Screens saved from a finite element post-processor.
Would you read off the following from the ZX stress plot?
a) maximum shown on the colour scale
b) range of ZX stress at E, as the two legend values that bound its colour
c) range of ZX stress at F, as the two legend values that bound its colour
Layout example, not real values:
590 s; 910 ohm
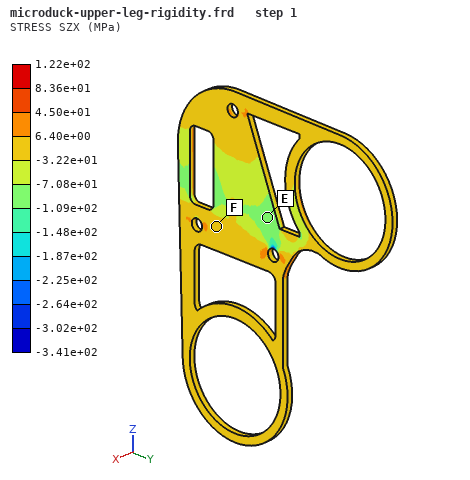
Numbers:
1.22e+02 MPa; -1.09e+02 to -7.08e+01 MPa; -3.22e+01 to 6.40e+00 MPa
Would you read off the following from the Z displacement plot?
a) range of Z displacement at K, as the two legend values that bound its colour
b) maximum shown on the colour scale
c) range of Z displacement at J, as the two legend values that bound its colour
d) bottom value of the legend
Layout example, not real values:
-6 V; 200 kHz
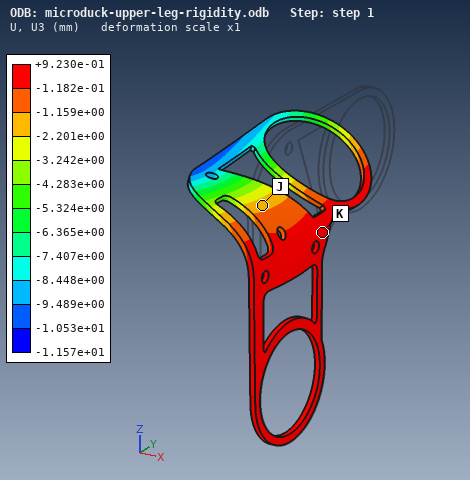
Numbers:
-1.182e-01 to +9.230e-01 mm; +9.230e-01 mm; -2.201e+00 to -1.159e+00 mm; -1.157e+01 mm
